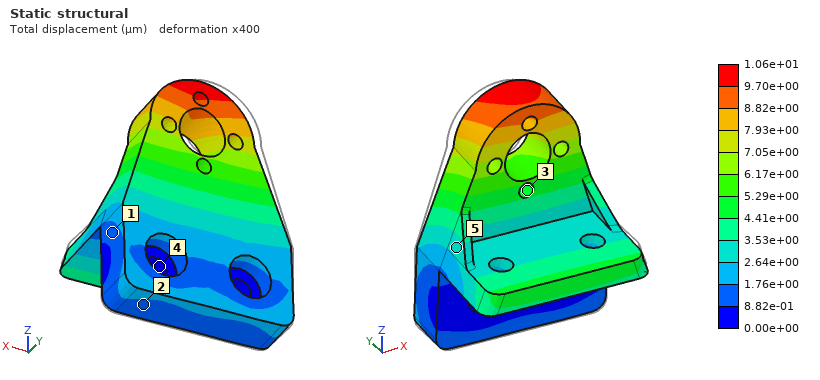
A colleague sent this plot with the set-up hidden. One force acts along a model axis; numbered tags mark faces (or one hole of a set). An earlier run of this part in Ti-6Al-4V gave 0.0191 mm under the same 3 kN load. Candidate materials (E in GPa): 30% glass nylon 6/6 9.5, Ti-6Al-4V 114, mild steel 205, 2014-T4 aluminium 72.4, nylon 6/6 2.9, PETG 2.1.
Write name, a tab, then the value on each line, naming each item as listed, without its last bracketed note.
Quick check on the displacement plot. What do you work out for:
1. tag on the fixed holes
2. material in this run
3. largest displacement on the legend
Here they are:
tag on the fixed holes	4
material in this run	mild steel
largest displacement on the legend	1.06e+01 µm
